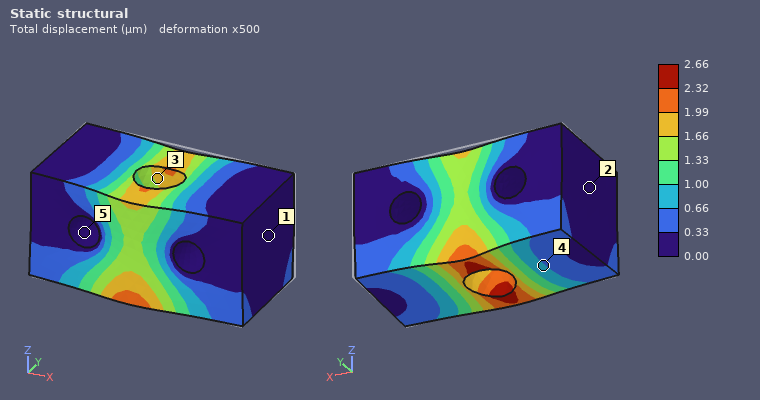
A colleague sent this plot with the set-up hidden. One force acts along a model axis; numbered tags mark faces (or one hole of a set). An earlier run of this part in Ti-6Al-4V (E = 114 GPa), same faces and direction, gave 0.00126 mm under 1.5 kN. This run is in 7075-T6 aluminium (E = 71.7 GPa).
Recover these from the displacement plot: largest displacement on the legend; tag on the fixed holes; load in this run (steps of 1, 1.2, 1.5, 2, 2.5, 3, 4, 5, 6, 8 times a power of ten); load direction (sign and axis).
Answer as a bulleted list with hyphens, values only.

- 2.66 µm
- 5
- 2 kN
- -Y
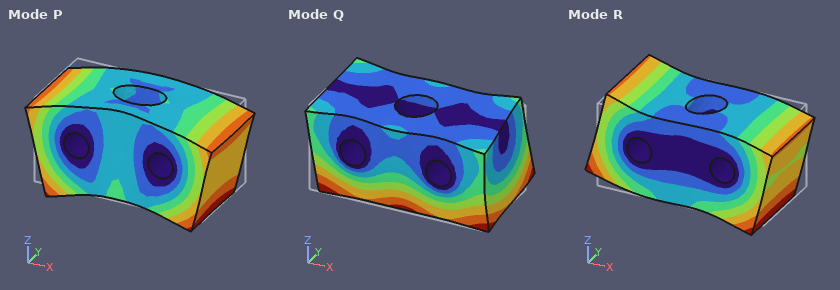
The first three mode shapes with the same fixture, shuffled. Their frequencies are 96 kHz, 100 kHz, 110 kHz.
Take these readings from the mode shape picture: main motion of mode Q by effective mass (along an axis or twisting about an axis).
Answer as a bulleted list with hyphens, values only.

- along Y
